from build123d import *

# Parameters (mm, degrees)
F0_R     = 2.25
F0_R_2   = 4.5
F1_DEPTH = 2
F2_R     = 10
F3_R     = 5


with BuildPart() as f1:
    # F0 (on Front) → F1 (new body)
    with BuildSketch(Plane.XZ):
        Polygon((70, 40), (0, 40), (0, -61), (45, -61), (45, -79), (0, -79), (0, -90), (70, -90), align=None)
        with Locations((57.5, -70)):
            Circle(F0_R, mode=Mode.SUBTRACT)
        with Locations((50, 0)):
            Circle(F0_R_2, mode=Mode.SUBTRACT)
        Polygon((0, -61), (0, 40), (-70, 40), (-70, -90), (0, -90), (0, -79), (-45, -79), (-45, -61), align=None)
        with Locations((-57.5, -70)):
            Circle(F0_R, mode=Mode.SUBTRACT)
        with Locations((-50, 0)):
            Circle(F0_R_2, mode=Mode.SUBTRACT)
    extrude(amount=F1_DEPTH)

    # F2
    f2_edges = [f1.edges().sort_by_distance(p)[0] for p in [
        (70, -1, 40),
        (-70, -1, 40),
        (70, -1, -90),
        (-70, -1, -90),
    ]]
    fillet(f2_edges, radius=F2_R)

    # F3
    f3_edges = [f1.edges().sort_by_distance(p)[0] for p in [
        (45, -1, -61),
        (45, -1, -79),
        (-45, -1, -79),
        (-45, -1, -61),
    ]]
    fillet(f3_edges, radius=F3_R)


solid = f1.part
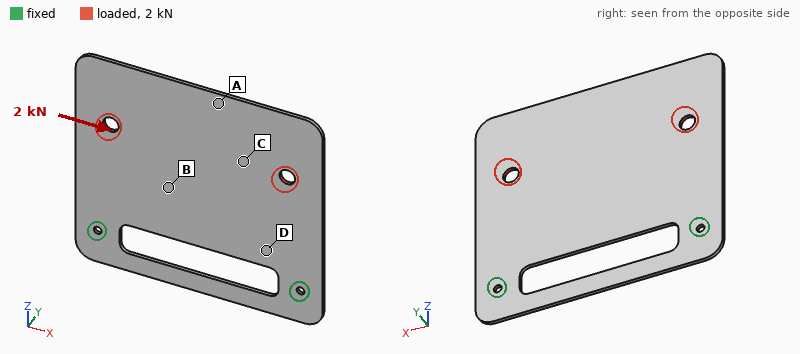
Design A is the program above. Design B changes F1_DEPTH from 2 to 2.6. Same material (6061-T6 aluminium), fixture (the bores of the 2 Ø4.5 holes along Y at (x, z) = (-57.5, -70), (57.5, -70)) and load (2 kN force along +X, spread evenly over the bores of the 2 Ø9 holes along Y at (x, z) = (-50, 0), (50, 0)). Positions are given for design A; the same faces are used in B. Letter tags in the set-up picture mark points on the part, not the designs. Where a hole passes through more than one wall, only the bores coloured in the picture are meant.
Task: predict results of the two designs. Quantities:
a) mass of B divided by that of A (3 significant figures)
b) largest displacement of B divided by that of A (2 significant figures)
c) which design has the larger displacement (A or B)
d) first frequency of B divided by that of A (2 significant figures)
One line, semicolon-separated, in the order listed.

1.30; 0.77; A; 1.3
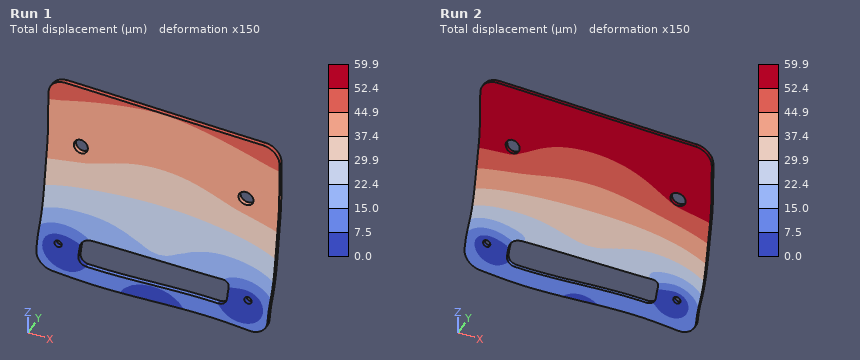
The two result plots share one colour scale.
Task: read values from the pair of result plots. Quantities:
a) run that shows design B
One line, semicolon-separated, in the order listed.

Run 1
